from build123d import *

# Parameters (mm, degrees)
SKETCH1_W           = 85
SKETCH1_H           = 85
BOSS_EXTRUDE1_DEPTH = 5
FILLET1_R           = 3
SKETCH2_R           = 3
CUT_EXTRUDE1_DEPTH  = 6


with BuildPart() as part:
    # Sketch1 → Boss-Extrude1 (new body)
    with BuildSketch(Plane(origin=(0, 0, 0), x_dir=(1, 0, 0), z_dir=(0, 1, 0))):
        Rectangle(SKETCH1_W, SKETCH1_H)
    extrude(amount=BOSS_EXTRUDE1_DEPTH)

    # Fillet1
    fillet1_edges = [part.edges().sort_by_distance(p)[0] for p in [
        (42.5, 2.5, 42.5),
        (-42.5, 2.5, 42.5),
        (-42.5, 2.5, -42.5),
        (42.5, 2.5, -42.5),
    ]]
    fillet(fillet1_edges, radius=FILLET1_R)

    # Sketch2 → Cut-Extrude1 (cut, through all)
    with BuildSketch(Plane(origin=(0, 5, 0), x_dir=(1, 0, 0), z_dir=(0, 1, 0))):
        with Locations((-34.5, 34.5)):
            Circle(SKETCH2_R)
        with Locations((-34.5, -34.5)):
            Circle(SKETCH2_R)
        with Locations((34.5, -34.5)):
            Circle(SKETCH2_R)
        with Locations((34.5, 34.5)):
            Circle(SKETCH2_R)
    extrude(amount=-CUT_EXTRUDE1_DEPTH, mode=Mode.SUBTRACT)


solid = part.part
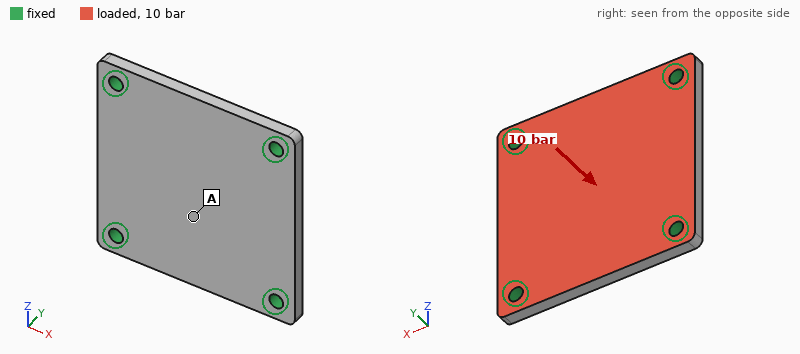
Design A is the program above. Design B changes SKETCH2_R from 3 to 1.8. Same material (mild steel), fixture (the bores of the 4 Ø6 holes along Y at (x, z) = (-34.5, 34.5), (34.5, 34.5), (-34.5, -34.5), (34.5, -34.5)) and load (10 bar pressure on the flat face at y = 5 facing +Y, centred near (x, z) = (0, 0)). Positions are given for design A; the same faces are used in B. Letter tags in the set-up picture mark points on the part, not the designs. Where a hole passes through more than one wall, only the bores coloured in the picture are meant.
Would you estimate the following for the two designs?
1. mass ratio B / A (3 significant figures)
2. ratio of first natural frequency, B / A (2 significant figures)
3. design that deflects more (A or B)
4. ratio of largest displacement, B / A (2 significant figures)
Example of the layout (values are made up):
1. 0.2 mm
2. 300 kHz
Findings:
1. 1.01
2. 0.91
3. B
4. 1.2
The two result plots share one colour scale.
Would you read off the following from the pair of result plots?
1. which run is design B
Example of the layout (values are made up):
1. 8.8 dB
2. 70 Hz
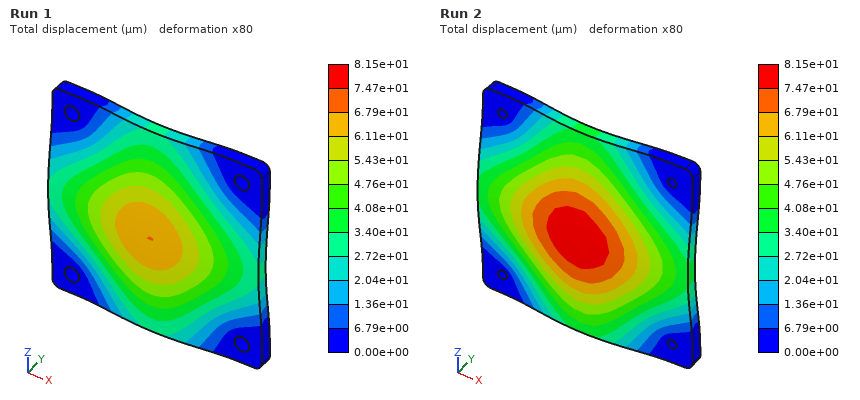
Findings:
1. Run 2
